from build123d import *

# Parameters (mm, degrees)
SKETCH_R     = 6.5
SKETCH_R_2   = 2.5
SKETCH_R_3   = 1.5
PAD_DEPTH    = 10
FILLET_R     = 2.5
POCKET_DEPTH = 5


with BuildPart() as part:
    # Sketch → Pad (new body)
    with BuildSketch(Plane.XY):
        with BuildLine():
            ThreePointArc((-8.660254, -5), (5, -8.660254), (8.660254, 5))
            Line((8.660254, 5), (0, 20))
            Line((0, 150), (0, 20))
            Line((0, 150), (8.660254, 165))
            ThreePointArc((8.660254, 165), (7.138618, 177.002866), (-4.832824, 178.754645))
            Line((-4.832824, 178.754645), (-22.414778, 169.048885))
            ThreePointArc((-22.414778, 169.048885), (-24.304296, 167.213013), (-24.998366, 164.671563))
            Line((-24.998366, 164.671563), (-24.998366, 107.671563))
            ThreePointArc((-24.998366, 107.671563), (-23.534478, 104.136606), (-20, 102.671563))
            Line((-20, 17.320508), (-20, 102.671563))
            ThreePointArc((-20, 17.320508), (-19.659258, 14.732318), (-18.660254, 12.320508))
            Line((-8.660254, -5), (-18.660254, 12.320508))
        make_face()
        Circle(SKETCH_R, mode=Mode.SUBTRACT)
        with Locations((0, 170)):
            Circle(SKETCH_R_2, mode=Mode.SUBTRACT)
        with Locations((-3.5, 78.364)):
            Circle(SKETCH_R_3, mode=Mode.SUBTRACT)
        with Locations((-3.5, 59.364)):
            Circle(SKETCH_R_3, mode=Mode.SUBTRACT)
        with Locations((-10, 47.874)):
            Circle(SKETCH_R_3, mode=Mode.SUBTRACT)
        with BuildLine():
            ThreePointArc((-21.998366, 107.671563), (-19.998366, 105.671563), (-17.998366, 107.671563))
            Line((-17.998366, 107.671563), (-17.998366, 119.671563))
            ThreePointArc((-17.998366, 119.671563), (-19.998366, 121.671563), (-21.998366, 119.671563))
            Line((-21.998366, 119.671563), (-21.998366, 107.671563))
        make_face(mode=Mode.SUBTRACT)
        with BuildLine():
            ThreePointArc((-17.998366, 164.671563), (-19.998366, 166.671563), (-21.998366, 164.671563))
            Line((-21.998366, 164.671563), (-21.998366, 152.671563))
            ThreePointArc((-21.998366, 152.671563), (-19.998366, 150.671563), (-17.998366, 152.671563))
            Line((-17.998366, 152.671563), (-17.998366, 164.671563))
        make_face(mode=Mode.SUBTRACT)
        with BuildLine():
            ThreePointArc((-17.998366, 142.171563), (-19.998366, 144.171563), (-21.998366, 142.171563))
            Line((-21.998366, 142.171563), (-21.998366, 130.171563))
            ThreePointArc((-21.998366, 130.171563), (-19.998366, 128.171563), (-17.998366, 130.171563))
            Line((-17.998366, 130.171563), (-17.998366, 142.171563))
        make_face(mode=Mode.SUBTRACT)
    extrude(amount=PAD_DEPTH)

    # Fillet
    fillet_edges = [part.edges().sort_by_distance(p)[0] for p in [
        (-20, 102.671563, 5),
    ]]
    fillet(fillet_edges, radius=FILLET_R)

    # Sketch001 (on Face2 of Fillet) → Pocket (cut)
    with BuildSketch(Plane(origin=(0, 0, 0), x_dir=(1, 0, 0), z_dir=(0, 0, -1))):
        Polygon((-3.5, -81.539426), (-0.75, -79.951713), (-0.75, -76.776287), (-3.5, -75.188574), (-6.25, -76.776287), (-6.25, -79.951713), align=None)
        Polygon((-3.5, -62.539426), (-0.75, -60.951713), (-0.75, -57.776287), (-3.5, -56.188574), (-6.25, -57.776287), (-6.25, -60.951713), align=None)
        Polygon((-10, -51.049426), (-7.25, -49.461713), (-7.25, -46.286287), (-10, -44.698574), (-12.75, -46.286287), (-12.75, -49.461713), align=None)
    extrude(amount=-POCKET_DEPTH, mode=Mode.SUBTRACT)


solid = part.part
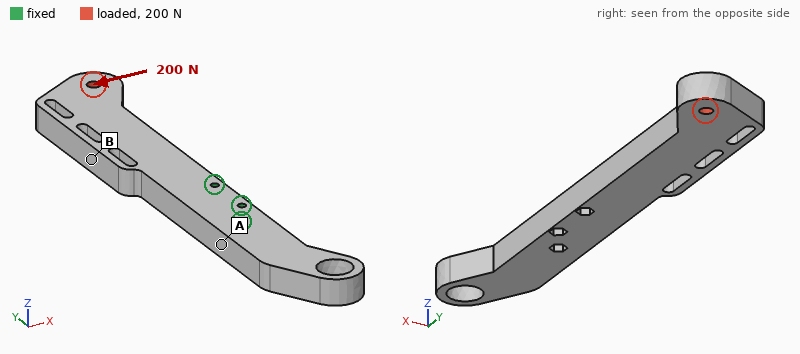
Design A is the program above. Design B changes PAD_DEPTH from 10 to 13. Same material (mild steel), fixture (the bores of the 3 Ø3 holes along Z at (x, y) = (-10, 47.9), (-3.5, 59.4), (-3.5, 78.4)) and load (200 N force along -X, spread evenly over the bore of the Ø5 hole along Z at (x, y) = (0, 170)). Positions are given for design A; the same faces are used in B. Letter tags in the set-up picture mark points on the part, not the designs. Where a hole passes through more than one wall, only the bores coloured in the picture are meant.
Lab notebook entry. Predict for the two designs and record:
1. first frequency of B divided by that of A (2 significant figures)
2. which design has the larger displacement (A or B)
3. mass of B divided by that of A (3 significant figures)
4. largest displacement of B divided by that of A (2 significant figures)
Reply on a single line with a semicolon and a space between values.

1.3; A; 1.30; 0.73
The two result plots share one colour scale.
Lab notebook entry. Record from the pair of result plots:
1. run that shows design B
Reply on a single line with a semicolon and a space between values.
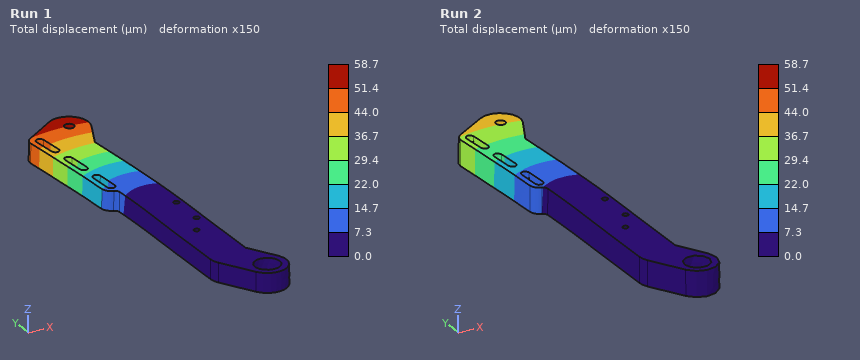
Run 2
